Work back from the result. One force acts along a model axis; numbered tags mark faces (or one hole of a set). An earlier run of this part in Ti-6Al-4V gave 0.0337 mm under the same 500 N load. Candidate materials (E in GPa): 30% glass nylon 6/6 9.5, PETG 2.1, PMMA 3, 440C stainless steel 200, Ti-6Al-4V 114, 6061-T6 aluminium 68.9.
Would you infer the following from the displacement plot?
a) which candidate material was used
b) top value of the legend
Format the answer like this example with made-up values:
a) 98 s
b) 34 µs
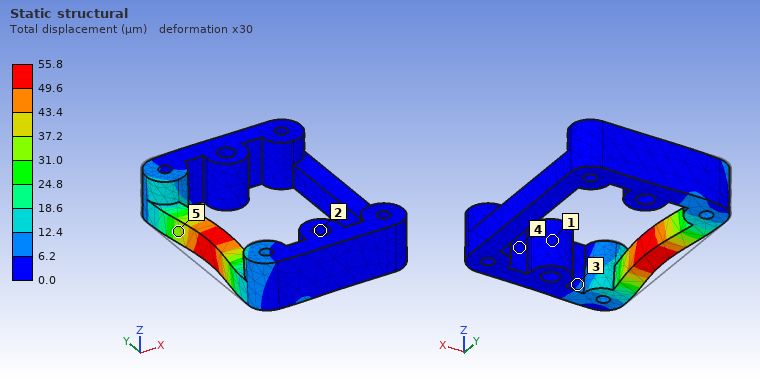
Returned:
a) 6061-T6 aluminium
b) 55.8 µm
